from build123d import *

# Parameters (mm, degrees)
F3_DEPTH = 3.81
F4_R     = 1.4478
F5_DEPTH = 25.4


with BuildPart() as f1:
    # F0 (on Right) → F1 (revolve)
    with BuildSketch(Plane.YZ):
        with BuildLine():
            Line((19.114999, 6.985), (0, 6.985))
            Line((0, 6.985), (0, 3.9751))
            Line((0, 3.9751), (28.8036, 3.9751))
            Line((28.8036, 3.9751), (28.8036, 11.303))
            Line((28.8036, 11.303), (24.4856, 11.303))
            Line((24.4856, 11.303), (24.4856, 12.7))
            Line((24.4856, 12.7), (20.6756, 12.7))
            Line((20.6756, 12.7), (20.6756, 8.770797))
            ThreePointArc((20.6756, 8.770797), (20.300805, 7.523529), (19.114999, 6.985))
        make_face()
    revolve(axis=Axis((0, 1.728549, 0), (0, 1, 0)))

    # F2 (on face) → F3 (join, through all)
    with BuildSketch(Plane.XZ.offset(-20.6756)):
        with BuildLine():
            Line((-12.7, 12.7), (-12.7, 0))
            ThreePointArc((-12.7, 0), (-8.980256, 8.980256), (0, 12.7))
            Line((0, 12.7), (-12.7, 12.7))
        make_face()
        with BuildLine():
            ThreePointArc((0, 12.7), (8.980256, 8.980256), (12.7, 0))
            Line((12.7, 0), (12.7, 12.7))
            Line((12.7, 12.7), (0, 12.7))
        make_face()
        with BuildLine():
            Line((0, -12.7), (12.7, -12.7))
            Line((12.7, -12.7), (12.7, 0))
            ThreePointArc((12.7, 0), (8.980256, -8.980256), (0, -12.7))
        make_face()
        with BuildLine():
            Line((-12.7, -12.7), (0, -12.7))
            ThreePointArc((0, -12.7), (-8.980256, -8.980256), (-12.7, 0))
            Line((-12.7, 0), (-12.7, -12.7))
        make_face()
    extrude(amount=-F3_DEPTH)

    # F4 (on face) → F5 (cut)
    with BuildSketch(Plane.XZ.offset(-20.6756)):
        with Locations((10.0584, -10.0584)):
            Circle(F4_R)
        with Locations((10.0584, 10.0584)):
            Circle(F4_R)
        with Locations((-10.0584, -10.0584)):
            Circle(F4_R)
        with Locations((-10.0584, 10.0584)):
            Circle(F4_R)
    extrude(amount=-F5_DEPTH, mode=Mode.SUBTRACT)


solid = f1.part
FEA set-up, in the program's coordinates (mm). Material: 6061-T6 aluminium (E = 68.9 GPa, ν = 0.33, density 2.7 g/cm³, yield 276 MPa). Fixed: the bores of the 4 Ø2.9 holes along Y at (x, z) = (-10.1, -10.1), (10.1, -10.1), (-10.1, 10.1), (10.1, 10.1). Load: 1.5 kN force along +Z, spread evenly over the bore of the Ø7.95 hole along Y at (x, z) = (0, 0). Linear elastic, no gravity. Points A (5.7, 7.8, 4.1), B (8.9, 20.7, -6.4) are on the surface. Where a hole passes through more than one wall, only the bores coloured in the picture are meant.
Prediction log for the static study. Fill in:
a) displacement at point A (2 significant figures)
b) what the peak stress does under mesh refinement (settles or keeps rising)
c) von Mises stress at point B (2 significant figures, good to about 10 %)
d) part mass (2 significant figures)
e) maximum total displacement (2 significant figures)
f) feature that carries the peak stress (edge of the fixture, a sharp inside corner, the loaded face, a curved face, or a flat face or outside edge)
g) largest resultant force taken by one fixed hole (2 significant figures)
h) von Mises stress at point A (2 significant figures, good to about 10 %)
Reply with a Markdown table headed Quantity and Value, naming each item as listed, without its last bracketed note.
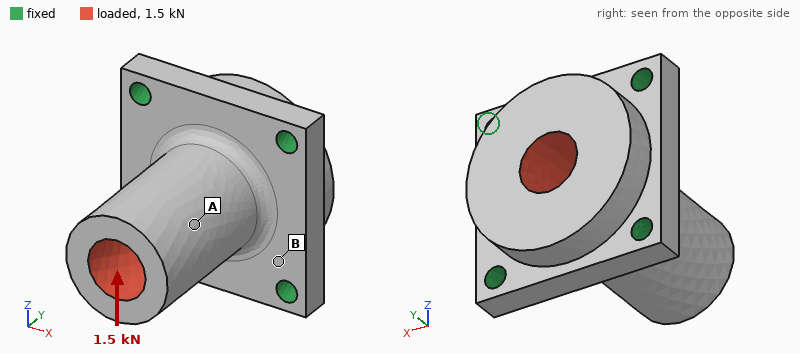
| Quantity | Value |
|---|---|
| displacement at point A | 22 µm |
| what the peak stress does under mesh refinement | keeps rising |
| von Mises stress at point B | 27 MPa |
| part mass | 16 g |
| maximum total displacement | 34 µm |
| feature that carries the peak stress | edge of the fixture |
| largest resultant force taken by one fixed hole | 510 N |
| von Mises stress at point A | 9.8 MPa |
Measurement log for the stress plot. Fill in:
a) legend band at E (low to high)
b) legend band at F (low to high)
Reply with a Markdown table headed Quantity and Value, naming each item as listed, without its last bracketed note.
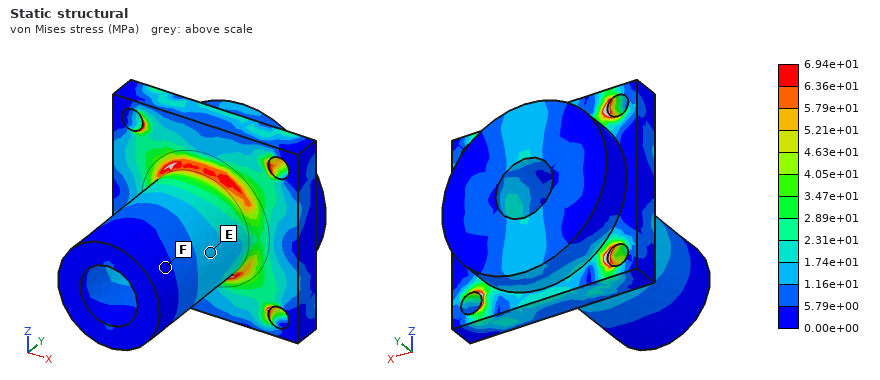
| Quantity | Value |
|---|---|
| legend band at E | 1.16e+01 to 1.74e+01 MPa |
| legend band at F | 0.00e+00 to 5.79e+00 MPa |
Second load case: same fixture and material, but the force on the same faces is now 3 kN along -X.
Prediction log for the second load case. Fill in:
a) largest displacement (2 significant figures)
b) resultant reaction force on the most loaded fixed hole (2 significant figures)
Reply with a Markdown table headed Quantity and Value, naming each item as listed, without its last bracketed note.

| Quantity | Value |
|---|---|
| largest displacement | 67 µm |
| resultant reaction force on the most loaded fixed hole | 1.0 kN |
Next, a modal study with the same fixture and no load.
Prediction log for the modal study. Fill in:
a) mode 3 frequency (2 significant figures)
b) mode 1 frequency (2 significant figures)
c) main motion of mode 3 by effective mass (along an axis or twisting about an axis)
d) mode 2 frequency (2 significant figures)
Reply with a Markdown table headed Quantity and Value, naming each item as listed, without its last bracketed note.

| Quantity | Value |
|---|---|
| mode 3 frequency | 26 kHz |
| mode 1 frequency | 14 kHz |
| main motion of mode 3 by effective mass | along Y |
| mode 2 frequency | 14 kHz |
